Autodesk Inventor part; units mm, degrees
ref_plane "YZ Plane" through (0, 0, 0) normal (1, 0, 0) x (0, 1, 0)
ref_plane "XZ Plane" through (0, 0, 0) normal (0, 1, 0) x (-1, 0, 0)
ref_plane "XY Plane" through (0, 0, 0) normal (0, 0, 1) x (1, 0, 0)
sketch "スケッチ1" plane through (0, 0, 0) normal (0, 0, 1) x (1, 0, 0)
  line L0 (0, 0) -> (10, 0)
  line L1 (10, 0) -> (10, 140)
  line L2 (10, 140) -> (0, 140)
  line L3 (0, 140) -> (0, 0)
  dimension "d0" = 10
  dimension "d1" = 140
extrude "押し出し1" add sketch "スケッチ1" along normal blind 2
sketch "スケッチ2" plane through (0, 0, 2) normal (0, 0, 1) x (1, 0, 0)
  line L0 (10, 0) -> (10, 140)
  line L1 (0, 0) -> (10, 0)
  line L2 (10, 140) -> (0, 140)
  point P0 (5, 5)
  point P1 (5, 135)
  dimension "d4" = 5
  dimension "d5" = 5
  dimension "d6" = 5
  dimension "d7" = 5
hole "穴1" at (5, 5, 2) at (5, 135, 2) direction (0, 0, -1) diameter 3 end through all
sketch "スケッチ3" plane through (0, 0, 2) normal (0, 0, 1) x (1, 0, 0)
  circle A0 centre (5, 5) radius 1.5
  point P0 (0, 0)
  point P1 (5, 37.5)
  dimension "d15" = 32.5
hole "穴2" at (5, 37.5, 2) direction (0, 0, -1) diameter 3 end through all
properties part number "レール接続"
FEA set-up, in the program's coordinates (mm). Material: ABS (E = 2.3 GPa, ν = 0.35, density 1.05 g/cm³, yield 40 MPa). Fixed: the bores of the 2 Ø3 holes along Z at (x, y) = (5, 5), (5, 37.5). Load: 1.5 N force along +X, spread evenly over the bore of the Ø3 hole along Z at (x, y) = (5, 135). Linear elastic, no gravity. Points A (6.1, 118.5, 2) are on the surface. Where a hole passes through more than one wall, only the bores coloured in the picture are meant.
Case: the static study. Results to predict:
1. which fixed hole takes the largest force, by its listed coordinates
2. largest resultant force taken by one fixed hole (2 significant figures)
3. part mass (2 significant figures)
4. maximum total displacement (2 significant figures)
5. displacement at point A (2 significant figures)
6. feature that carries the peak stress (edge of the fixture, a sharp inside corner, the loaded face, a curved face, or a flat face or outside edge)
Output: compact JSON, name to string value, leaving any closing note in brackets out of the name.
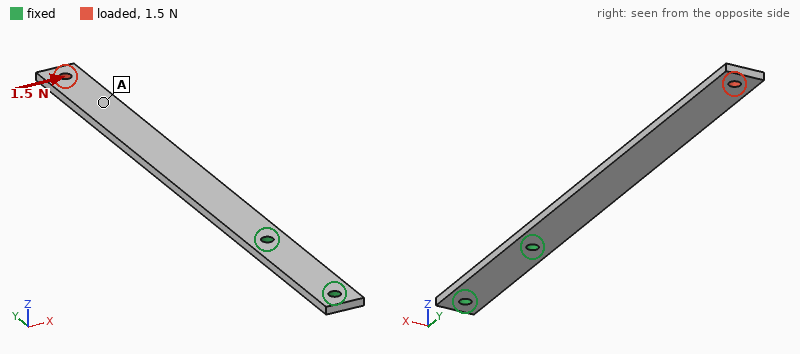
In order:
{"which fixed hole takes the largest force, by its listed coordinates": "(5, 37.5)", "largest resultant force taken by one fixed hole": "3.7 N", "part mass": "2.9 g", "maximum total displacement": "1.5 mm", "displacement at point A": "1.0 mm", "feature that carries the peak stress": "edge of the fixture"}
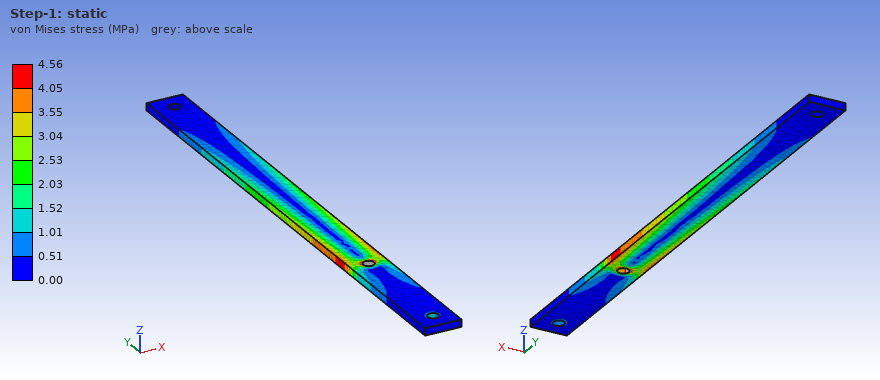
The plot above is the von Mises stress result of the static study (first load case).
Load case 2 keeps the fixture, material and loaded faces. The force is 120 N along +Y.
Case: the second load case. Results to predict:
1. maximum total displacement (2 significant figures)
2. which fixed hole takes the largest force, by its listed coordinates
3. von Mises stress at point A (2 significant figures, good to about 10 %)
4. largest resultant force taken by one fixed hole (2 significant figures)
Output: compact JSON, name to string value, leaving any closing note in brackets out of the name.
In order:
{"maximum total displacement": "0.27 mm", "which fixed hole takes the largest force, by its listed coordinates": "(5, 37.5)", "von Mises stress at point A": "6.0 MPa", "largest resultant force taken by one fixed hole": "120 N"}
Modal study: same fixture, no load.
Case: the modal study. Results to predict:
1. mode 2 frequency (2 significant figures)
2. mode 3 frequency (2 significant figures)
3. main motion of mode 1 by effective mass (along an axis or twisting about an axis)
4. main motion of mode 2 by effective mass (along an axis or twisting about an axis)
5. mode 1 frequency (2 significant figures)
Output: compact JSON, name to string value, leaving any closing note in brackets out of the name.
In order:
{"mode 2 frequency": "210 Hz", "mode 3 frequency": "290 Hz", "main motion of mode 1 by effective mass": "along Z", "main motion of mode 2 by effective mass": "along X", "mode 1 frequency": "47 Hz"}
